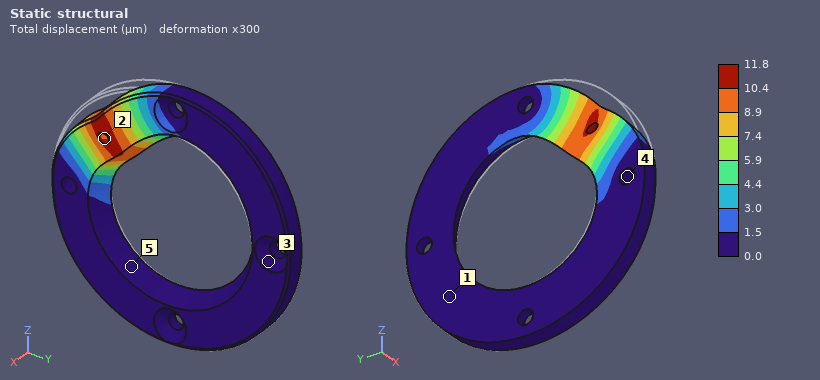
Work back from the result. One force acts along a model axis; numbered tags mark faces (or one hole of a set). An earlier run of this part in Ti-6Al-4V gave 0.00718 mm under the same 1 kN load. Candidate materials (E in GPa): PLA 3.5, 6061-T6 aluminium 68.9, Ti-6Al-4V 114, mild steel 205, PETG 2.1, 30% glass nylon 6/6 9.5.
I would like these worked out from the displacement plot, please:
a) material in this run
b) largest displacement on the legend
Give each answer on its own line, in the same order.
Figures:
6061-T6 aluminium
11.8 µm
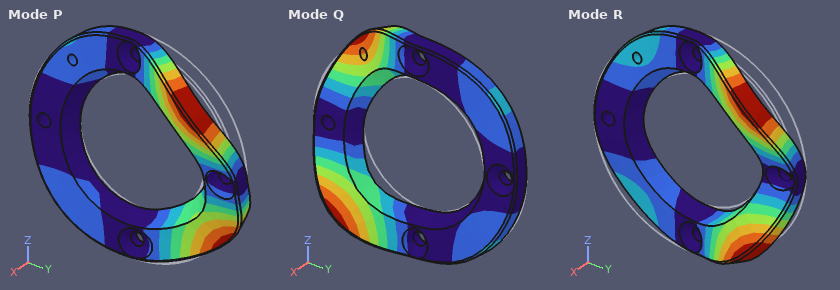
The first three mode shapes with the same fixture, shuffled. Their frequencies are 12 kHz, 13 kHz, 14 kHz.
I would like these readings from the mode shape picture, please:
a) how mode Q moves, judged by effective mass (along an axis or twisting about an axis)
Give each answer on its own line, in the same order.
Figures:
twisting about Y
